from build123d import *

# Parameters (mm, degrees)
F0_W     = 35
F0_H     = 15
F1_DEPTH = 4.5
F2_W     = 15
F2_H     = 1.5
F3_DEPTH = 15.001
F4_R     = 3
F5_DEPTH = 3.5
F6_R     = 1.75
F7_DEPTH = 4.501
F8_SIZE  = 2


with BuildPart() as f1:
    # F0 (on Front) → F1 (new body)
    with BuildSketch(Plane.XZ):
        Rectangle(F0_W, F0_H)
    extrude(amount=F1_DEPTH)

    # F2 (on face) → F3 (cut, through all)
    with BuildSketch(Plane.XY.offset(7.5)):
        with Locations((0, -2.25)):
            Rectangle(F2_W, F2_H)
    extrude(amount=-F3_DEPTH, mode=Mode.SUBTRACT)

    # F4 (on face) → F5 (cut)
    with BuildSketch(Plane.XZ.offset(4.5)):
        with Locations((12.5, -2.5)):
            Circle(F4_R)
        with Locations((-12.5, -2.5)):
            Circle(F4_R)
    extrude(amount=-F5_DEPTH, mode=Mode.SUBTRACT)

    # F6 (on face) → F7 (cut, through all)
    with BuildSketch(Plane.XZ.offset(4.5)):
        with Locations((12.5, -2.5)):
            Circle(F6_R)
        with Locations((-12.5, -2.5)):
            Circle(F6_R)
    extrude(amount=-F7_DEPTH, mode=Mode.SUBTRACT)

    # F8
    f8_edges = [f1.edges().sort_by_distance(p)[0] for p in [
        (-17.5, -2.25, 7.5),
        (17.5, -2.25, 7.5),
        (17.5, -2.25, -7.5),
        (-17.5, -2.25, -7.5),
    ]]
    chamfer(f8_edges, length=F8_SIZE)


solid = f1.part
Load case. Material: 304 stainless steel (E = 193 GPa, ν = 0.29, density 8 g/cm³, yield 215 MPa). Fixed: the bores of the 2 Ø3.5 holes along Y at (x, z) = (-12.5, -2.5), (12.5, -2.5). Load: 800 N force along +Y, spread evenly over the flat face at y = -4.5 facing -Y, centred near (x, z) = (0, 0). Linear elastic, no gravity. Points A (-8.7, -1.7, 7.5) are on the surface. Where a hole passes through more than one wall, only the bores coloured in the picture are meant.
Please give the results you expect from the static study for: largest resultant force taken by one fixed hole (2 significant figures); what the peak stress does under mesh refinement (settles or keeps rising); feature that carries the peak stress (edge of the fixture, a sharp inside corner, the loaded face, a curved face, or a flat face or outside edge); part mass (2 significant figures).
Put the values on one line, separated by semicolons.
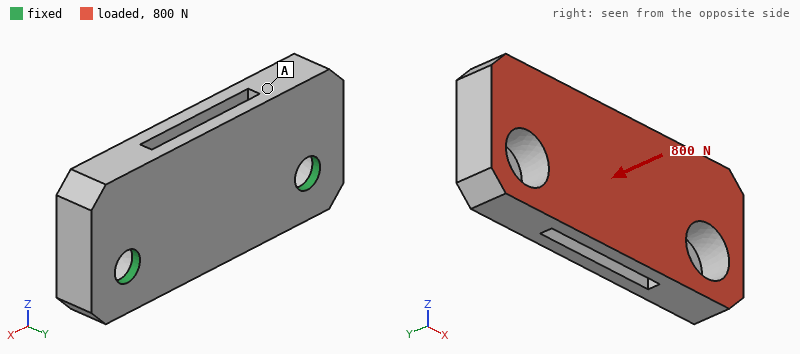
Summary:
450 N; keeps rising; edge of the fixture; 14 g
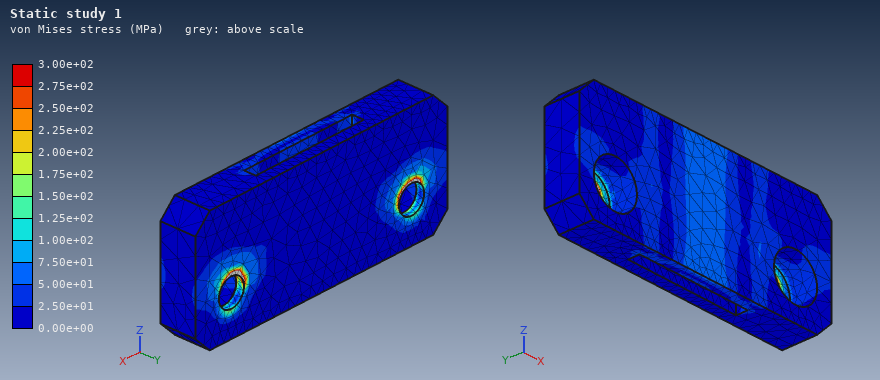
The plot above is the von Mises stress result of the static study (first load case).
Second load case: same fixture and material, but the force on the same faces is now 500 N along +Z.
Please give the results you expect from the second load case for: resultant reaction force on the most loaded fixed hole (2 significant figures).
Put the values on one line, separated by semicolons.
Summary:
250 N
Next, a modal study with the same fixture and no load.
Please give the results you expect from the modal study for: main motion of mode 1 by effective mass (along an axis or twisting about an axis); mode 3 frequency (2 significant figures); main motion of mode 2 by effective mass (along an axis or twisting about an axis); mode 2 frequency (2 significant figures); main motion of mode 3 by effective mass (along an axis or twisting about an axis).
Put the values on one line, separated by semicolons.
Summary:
along Y; 19 kHz; twisting about Z; 16 kHz; along Y
